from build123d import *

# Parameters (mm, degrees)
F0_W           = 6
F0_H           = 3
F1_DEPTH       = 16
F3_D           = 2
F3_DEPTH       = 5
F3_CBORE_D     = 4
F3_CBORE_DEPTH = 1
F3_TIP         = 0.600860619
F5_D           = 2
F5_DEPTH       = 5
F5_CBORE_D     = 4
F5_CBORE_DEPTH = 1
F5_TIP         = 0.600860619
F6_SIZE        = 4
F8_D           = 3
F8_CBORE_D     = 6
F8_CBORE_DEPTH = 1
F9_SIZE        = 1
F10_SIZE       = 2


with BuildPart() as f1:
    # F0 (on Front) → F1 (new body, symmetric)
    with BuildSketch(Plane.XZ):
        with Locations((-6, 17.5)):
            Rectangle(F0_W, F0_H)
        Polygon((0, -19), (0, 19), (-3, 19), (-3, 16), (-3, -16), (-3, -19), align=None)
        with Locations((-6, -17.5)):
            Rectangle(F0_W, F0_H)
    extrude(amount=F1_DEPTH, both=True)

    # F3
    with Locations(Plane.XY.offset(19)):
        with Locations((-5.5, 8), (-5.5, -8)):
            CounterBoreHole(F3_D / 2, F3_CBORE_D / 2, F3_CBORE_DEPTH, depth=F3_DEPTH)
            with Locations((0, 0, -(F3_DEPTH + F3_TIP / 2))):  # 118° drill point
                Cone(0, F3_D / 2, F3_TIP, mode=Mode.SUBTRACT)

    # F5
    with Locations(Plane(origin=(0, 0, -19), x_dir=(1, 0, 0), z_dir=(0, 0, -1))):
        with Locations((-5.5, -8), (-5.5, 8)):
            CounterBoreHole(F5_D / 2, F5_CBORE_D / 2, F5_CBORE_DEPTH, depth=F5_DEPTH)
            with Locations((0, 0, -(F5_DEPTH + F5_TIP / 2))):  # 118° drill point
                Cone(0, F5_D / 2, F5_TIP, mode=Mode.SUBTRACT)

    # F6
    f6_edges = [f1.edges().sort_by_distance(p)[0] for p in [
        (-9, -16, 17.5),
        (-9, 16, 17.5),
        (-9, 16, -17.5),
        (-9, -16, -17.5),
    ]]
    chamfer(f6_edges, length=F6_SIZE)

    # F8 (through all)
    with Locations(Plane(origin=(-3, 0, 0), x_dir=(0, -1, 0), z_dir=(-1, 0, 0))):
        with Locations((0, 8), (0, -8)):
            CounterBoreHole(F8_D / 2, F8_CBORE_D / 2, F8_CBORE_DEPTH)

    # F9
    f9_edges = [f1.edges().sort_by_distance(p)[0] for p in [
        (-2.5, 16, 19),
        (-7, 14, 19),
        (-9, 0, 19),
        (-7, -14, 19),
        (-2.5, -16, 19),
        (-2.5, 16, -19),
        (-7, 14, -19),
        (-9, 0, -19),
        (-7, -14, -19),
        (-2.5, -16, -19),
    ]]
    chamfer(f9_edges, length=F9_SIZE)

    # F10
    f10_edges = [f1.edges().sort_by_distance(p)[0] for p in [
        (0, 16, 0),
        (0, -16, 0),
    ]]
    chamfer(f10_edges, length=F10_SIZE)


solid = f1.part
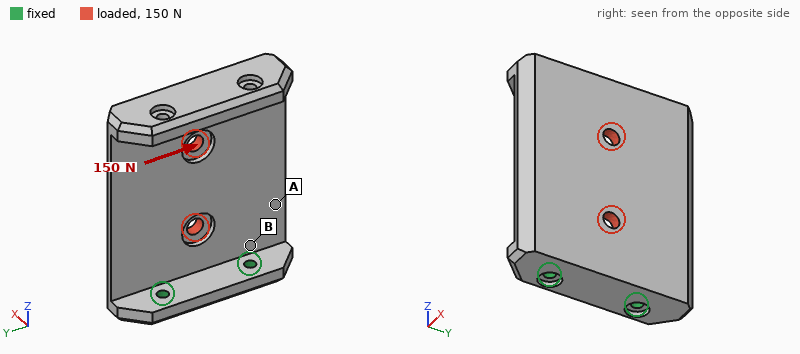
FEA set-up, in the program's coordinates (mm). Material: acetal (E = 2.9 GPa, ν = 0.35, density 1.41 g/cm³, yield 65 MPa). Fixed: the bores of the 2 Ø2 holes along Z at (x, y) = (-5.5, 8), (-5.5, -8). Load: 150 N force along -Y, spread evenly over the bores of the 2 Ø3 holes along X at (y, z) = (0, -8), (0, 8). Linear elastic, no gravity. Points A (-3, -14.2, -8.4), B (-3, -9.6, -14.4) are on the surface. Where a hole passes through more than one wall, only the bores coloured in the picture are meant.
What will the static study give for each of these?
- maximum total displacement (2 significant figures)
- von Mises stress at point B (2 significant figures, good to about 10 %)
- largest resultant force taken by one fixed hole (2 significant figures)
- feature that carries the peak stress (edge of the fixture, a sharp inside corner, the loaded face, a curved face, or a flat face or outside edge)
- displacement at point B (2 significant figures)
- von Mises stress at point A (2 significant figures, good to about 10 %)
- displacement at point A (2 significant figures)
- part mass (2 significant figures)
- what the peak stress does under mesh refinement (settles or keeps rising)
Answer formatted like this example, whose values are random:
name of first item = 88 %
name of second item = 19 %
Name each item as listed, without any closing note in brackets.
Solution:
maximum total displacement = 0.50 mm
von Mises stress at point B = 14 MPa
largest resultant force taken by one fixed hole = 170 N
feature that carries the peak stress = edge of the fixture
displacement at point B = 0.090 mm
von Mises stress at point A = 5.7 MPa
displacement at point A = 0.21 mm
part mass = 6.1 g
what the peak stress does under mesh refinement = keeps rising
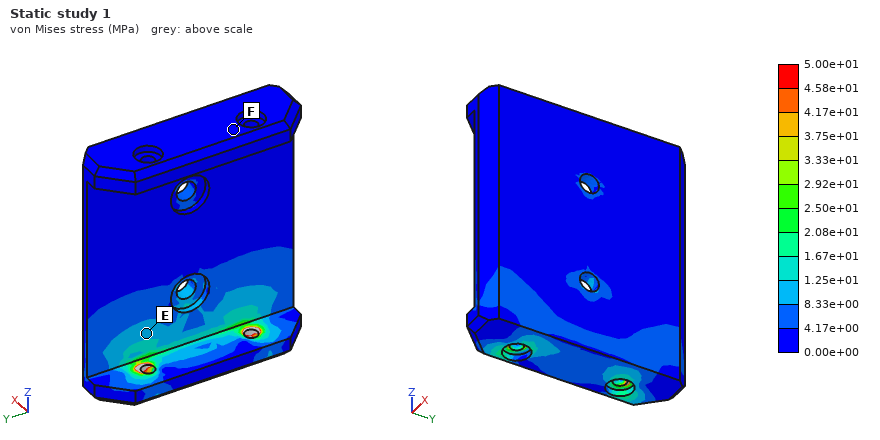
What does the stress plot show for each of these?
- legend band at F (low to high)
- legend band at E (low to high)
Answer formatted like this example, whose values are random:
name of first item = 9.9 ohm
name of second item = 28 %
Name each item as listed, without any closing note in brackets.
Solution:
legend band at F = 0.00e+00 to 4.17e+00 MPa
legend band at E = 8.33e+00 to 1.25e+01 MPa
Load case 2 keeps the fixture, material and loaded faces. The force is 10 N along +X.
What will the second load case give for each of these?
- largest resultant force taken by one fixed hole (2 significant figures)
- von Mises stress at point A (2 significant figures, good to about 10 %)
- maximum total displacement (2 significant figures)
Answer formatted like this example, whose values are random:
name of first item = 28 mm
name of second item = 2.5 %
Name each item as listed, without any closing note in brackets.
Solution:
largest resultant force taken by one fixed hole = 5.1 N
von Mises stress at point A = 2.0 MPa
maximum total displacement = 0.52 mm
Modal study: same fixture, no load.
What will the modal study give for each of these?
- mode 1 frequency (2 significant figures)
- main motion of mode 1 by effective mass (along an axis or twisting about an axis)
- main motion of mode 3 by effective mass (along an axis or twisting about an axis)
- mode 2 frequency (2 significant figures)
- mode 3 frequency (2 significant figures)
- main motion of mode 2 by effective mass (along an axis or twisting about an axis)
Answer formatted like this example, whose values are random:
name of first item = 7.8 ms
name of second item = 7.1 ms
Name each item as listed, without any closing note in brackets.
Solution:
mode 1 frequency = 320 Hz
main motion of mode 1 by effective mass = along X
main motion of mode 3 by effective mass = along Y
mode 2 frequency = 970 Hz
mode 3 frequency = 1500 Hz
main motion of mode 2 by effective mass = along Y
